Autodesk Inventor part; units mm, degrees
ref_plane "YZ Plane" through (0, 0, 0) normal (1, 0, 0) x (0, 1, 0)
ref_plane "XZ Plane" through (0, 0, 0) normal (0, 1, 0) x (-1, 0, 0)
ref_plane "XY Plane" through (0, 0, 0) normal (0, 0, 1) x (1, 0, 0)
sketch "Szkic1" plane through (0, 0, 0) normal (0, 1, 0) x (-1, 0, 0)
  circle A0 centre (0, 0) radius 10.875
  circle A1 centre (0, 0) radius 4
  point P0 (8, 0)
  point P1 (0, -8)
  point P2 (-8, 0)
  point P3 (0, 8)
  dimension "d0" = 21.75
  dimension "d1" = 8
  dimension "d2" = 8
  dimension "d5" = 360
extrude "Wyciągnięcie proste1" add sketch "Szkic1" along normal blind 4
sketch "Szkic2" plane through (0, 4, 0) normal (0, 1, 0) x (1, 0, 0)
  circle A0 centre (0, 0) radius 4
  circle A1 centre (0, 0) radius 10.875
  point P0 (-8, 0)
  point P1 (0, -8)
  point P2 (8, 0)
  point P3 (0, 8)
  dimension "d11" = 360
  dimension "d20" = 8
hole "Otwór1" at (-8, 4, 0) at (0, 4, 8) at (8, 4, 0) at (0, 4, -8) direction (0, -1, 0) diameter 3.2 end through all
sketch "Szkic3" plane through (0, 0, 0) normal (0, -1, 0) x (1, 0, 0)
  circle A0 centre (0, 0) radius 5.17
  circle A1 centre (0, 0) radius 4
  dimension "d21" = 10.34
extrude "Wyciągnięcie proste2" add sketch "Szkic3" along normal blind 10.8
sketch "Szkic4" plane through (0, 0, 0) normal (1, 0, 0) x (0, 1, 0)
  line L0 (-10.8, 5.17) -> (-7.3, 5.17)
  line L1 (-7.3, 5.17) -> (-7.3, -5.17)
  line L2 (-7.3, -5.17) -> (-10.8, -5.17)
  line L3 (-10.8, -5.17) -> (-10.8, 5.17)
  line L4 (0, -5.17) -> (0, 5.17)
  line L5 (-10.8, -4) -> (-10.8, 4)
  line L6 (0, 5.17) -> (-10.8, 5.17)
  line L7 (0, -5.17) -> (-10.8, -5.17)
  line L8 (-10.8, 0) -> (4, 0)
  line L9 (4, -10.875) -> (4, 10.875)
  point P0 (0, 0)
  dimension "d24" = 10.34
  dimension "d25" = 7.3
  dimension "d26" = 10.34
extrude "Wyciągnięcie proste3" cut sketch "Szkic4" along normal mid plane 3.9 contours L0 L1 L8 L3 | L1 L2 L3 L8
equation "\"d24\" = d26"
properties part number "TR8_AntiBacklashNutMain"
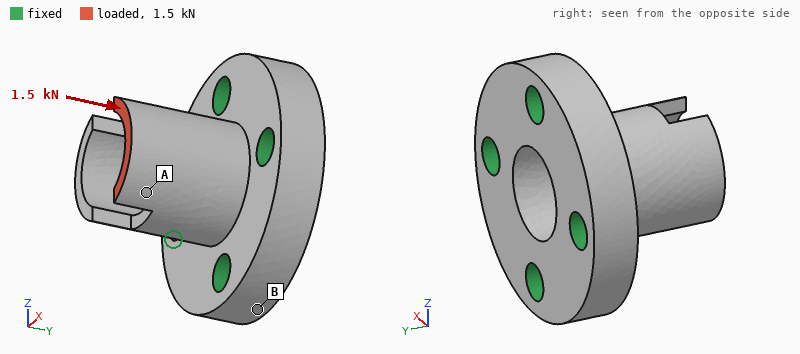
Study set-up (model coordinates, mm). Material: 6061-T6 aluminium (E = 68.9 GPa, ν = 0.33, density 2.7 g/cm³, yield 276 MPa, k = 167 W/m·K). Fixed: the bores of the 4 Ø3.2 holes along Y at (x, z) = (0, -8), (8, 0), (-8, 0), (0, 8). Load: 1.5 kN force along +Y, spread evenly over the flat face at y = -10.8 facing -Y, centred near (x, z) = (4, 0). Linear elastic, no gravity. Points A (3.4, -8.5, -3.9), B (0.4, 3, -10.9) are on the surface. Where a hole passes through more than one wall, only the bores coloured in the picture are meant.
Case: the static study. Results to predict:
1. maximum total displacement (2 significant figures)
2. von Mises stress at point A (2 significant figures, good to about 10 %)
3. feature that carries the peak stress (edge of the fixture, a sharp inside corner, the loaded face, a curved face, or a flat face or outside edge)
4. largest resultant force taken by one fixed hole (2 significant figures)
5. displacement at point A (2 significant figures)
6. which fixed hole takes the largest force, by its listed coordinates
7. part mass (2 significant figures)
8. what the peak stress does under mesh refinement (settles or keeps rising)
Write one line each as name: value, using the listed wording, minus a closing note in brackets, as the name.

maximum total displacement: 39 µm
von Mises stress at point A: 120 MPa
feature that carries the peak stress: edge of the fixture
largest resultant force taken by one fixed hole: 840 N
displacement at point A: 24 µm
which fixed hole takes the largest force, by its listed coordinates: (8, 0)
part mass: 4.0 g
what the peak stress does under mesh refinement: keeps rising
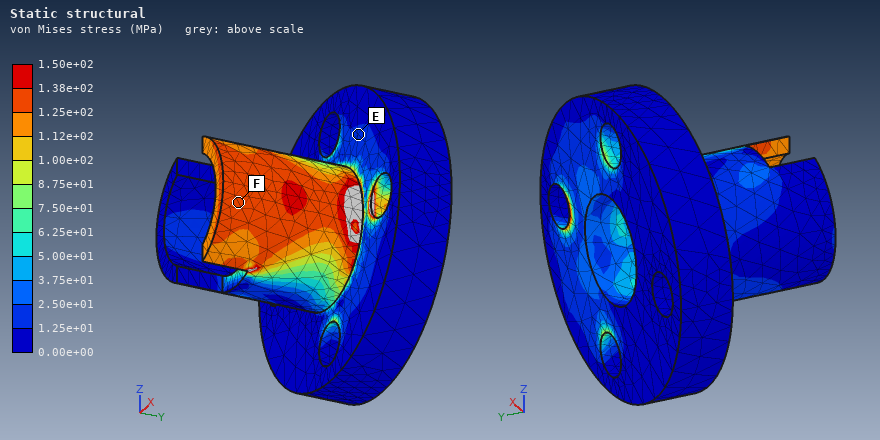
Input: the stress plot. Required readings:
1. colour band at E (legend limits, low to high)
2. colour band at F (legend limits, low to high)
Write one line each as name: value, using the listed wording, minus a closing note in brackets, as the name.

colour band at E: 1.25e+01 to 2.50e+01 MPa
colour band at F: 1.25e+02 to 1.38e+02 MPa
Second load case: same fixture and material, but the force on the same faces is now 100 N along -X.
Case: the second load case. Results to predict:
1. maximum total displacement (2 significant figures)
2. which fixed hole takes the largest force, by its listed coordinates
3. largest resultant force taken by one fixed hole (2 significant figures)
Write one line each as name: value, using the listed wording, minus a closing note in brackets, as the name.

maximum total displacement: 25 µm
which fixed hole takes the largest force, by its listed coordinates: (8, 0)
largest resultant force taken by one fixed hole: 130 N
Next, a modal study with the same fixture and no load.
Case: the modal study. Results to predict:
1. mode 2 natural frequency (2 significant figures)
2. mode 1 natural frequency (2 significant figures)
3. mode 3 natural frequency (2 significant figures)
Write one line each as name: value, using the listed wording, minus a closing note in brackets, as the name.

mode 2 natural frequency: 37 kHz
mode 1 natural frequency: 33 kHz
mode 3 natural frequency: 37 kHz
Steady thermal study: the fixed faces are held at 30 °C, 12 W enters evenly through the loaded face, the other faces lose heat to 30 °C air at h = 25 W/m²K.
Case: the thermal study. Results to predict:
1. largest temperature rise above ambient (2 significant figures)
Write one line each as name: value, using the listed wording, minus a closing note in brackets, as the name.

largest temperature rise above ambient: 52 K
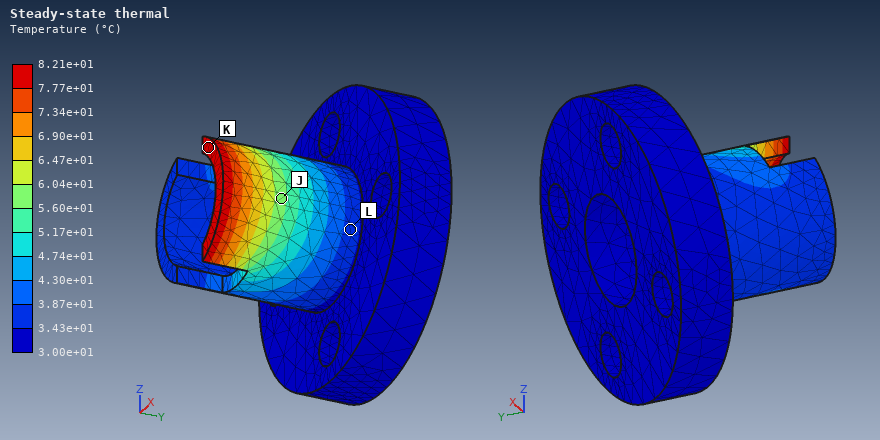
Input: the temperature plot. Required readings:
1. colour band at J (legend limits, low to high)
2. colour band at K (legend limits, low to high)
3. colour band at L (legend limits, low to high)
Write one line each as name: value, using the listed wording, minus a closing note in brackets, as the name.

colour band at J: 5.60e+01 to 6.04e+01 °C
colour band at K: 7.77e+01 to 8.21e+01 °C
colour band at L: 3.43e+01 to 3.87e+01 °C
